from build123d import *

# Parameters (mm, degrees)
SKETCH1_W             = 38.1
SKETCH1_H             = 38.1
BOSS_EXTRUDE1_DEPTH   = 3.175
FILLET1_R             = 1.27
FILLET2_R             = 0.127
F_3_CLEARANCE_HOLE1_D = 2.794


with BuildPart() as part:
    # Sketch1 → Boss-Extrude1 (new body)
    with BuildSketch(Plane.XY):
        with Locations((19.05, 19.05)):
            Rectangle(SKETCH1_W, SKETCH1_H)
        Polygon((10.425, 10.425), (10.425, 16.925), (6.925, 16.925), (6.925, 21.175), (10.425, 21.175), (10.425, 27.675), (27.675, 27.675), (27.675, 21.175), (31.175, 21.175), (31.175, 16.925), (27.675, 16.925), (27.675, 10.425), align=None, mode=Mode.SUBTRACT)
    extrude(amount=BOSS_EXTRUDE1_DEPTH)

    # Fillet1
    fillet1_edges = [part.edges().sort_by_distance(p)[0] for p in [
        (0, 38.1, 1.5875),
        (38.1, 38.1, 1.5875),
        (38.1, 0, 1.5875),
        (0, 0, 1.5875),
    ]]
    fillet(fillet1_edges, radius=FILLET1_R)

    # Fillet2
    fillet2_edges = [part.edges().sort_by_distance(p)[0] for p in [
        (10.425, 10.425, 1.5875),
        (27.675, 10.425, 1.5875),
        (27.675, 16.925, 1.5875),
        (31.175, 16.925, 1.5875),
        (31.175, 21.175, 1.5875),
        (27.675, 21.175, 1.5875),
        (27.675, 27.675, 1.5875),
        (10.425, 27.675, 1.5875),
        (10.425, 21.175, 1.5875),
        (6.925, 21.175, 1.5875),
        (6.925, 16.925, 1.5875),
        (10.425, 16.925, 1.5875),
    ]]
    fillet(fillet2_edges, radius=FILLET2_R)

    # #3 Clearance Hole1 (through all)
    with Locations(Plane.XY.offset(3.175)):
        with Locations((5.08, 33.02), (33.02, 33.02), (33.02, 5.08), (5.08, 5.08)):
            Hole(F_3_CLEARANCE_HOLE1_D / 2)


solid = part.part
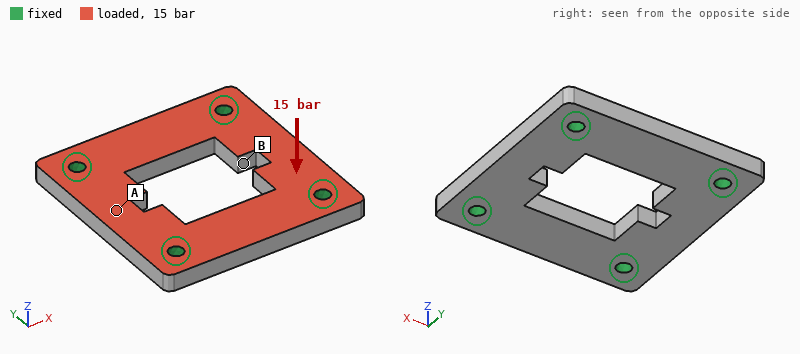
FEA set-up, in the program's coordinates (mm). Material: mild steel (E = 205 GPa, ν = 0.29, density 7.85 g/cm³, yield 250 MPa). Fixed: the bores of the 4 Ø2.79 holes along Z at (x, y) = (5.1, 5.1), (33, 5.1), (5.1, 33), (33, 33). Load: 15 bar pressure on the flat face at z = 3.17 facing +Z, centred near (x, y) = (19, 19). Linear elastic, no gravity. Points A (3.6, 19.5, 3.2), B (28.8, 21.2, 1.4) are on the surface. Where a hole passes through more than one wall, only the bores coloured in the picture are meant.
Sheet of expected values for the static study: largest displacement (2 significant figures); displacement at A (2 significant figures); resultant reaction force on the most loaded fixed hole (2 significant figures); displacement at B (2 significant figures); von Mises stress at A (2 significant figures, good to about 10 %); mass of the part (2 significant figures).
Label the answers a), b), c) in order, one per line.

a) 5.9 µm
b) 4.4 µm
c) 410 N
d) 5.6 µm
e) 28 MPa
f) 27 g
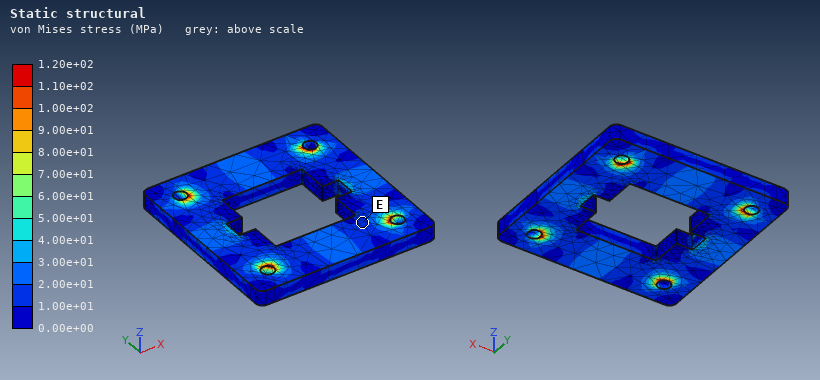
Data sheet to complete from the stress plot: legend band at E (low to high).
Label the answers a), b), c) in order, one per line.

a) 1.00e+01 to 2.00e+01 MPa
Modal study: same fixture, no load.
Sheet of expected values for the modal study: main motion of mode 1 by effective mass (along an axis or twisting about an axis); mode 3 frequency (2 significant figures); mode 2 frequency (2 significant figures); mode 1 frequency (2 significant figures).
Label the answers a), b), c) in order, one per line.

a) along Z
b) 21 kHz
c) 21 kHz
d) 20 kHz
